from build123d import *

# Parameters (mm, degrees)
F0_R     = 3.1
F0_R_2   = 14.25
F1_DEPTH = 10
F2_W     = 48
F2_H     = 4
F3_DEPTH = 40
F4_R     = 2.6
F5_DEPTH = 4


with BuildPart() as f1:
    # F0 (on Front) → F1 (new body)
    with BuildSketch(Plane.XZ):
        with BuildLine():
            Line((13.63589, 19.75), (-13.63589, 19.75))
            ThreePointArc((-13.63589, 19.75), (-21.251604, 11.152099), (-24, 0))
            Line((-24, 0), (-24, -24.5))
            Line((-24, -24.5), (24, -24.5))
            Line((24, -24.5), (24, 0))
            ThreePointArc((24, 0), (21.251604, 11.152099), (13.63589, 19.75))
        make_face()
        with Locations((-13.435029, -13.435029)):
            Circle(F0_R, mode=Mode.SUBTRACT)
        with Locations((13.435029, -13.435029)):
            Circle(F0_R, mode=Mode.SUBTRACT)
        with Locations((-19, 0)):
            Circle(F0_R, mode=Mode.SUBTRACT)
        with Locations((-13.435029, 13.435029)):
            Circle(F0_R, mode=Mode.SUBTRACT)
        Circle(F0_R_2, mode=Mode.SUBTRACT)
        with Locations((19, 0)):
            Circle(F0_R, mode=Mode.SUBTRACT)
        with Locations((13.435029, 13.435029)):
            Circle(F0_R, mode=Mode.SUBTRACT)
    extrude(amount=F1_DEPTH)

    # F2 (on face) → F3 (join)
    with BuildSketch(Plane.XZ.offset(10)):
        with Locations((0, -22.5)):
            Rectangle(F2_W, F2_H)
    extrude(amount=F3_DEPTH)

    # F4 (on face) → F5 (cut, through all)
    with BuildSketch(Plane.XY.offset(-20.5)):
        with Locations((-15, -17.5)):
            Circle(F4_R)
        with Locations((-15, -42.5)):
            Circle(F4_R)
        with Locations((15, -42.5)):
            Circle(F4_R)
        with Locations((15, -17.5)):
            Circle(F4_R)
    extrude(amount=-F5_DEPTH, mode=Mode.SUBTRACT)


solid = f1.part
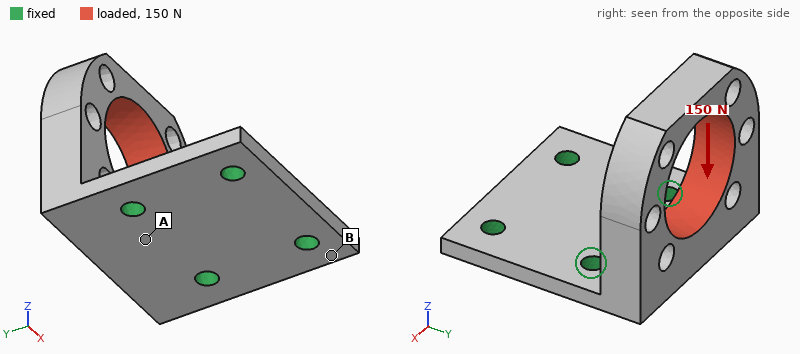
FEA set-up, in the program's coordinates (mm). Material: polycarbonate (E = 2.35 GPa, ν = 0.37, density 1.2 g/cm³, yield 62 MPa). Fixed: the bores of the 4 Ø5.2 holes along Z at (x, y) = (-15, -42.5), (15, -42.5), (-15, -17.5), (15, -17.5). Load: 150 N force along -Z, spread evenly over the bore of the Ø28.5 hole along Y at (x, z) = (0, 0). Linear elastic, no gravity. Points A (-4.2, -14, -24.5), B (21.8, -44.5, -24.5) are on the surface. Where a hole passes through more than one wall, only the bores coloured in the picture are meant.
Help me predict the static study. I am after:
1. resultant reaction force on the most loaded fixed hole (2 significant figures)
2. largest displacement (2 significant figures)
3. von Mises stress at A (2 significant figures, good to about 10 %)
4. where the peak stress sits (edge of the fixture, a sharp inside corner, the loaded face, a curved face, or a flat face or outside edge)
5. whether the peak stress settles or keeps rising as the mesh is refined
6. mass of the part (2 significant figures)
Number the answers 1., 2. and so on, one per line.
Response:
1. 81 N
2. 0.72 mm
3. 5.2 MPa
4. edge of the fixture
5. keeps rising
6. 23 g
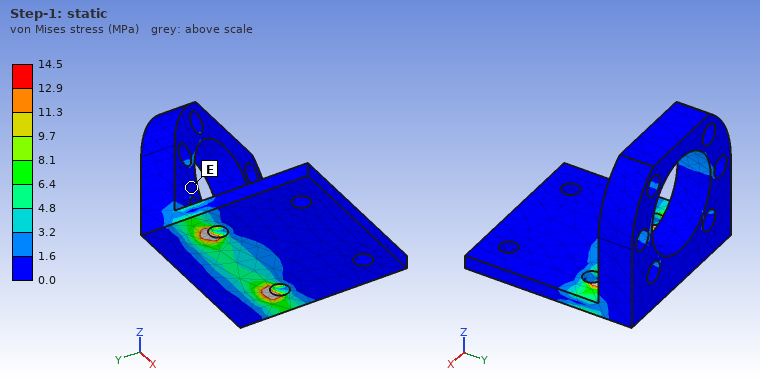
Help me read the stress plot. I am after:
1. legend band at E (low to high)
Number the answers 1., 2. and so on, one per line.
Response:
1. 0.0 to 1.6 MPa
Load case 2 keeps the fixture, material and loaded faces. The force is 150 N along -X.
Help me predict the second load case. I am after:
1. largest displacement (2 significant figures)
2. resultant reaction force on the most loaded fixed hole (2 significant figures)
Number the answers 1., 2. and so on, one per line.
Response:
1. 0.31 mm
2. 140 N
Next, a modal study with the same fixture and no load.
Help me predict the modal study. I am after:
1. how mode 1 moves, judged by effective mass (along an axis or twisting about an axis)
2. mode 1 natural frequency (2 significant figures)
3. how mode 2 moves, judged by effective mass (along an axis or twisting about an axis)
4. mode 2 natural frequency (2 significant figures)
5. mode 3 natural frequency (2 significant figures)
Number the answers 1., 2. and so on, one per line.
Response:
1. along Y
2. 450 Hz
3. along X
4. 1100 Hz
5. 1800 Hz
